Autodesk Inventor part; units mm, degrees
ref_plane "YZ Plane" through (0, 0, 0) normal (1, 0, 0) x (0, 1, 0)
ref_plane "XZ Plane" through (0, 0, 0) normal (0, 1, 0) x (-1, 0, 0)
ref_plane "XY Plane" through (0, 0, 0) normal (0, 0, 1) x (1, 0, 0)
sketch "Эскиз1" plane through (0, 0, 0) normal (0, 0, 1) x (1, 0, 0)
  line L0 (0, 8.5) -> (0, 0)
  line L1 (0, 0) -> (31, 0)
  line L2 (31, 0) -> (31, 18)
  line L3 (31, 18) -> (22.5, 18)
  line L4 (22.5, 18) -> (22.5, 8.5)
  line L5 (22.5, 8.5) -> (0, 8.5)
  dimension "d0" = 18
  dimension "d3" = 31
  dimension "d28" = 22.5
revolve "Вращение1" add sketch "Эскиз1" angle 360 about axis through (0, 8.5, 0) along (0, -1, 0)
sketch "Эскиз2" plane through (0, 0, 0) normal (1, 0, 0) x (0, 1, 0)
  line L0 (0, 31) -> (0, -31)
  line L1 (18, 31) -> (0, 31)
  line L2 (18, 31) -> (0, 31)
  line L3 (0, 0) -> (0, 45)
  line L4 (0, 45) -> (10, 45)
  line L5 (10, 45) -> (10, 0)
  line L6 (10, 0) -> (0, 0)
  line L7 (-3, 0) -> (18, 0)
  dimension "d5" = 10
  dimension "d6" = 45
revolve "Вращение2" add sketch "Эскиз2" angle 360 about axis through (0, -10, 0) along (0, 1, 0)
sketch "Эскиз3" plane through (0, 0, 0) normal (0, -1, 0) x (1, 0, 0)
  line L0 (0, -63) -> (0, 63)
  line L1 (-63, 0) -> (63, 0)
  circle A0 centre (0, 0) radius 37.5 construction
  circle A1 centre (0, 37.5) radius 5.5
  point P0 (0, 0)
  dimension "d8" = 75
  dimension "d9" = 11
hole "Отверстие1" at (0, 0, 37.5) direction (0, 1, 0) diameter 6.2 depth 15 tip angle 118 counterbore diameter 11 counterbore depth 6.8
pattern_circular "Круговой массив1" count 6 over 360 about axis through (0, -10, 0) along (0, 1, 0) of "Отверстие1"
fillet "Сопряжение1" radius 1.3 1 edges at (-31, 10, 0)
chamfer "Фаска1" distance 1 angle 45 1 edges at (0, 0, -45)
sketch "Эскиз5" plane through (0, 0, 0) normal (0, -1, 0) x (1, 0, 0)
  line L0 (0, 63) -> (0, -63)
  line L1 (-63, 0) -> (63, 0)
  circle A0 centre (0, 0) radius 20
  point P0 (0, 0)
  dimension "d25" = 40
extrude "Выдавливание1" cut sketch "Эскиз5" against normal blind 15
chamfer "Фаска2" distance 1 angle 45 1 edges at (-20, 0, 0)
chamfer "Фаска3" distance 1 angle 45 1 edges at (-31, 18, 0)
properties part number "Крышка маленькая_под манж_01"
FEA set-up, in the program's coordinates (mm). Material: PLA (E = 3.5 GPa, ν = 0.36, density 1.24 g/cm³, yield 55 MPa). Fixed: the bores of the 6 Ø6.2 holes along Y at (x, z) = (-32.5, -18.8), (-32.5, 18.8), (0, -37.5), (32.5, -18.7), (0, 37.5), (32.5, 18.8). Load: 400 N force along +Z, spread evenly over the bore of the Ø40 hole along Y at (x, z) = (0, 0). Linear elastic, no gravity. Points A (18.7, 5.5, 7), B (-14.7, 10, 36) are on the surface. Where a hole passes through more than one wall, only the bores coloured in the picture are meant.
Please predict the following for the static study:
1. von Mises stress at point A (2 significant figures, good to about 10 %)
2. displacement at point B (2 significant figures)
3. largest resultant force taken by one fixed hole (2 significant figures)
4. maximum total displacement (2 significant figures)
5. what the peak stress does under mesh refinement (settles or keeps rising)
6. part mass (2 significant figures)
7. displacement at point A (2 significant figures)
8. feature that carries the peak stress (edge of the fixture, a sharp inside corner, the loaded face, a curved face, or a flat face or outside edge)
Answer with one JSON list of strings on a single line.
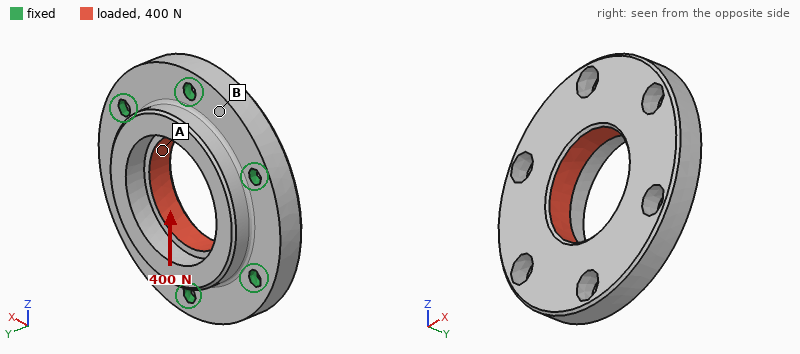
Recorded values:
["0.56 MPa", "2.8 µm", "84 N", "5.3 µm", "keeps rising", "72 g", "4.1 µm", "edge of the fixture"]
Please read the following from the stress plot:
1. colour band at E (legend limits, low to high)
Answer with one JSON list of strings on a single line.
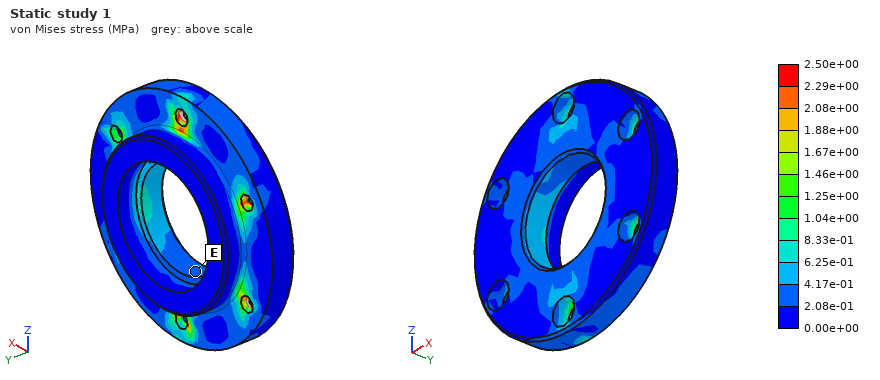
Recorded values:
["2.08e-01 to 4.17e-01 MPa"]
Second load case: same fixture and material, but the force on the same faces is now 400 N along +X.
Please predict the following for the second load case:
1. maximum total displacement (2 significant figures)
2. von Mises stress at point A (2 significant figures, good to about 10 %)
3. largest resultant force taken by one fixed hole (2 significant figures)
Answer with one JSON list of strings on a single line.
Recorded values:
["5.5 µm", "0.33 MPa", "77 N"]
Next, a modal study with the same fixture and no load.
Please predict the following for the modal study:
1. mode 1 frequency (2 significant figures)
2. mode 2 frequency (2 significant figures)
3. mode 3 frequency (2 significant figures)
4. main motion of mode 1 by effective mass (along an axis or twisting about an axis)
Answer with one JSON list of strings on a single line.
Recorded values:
["4400 Hz", "5700 Hz", "5700 Hz", "along Y"]
